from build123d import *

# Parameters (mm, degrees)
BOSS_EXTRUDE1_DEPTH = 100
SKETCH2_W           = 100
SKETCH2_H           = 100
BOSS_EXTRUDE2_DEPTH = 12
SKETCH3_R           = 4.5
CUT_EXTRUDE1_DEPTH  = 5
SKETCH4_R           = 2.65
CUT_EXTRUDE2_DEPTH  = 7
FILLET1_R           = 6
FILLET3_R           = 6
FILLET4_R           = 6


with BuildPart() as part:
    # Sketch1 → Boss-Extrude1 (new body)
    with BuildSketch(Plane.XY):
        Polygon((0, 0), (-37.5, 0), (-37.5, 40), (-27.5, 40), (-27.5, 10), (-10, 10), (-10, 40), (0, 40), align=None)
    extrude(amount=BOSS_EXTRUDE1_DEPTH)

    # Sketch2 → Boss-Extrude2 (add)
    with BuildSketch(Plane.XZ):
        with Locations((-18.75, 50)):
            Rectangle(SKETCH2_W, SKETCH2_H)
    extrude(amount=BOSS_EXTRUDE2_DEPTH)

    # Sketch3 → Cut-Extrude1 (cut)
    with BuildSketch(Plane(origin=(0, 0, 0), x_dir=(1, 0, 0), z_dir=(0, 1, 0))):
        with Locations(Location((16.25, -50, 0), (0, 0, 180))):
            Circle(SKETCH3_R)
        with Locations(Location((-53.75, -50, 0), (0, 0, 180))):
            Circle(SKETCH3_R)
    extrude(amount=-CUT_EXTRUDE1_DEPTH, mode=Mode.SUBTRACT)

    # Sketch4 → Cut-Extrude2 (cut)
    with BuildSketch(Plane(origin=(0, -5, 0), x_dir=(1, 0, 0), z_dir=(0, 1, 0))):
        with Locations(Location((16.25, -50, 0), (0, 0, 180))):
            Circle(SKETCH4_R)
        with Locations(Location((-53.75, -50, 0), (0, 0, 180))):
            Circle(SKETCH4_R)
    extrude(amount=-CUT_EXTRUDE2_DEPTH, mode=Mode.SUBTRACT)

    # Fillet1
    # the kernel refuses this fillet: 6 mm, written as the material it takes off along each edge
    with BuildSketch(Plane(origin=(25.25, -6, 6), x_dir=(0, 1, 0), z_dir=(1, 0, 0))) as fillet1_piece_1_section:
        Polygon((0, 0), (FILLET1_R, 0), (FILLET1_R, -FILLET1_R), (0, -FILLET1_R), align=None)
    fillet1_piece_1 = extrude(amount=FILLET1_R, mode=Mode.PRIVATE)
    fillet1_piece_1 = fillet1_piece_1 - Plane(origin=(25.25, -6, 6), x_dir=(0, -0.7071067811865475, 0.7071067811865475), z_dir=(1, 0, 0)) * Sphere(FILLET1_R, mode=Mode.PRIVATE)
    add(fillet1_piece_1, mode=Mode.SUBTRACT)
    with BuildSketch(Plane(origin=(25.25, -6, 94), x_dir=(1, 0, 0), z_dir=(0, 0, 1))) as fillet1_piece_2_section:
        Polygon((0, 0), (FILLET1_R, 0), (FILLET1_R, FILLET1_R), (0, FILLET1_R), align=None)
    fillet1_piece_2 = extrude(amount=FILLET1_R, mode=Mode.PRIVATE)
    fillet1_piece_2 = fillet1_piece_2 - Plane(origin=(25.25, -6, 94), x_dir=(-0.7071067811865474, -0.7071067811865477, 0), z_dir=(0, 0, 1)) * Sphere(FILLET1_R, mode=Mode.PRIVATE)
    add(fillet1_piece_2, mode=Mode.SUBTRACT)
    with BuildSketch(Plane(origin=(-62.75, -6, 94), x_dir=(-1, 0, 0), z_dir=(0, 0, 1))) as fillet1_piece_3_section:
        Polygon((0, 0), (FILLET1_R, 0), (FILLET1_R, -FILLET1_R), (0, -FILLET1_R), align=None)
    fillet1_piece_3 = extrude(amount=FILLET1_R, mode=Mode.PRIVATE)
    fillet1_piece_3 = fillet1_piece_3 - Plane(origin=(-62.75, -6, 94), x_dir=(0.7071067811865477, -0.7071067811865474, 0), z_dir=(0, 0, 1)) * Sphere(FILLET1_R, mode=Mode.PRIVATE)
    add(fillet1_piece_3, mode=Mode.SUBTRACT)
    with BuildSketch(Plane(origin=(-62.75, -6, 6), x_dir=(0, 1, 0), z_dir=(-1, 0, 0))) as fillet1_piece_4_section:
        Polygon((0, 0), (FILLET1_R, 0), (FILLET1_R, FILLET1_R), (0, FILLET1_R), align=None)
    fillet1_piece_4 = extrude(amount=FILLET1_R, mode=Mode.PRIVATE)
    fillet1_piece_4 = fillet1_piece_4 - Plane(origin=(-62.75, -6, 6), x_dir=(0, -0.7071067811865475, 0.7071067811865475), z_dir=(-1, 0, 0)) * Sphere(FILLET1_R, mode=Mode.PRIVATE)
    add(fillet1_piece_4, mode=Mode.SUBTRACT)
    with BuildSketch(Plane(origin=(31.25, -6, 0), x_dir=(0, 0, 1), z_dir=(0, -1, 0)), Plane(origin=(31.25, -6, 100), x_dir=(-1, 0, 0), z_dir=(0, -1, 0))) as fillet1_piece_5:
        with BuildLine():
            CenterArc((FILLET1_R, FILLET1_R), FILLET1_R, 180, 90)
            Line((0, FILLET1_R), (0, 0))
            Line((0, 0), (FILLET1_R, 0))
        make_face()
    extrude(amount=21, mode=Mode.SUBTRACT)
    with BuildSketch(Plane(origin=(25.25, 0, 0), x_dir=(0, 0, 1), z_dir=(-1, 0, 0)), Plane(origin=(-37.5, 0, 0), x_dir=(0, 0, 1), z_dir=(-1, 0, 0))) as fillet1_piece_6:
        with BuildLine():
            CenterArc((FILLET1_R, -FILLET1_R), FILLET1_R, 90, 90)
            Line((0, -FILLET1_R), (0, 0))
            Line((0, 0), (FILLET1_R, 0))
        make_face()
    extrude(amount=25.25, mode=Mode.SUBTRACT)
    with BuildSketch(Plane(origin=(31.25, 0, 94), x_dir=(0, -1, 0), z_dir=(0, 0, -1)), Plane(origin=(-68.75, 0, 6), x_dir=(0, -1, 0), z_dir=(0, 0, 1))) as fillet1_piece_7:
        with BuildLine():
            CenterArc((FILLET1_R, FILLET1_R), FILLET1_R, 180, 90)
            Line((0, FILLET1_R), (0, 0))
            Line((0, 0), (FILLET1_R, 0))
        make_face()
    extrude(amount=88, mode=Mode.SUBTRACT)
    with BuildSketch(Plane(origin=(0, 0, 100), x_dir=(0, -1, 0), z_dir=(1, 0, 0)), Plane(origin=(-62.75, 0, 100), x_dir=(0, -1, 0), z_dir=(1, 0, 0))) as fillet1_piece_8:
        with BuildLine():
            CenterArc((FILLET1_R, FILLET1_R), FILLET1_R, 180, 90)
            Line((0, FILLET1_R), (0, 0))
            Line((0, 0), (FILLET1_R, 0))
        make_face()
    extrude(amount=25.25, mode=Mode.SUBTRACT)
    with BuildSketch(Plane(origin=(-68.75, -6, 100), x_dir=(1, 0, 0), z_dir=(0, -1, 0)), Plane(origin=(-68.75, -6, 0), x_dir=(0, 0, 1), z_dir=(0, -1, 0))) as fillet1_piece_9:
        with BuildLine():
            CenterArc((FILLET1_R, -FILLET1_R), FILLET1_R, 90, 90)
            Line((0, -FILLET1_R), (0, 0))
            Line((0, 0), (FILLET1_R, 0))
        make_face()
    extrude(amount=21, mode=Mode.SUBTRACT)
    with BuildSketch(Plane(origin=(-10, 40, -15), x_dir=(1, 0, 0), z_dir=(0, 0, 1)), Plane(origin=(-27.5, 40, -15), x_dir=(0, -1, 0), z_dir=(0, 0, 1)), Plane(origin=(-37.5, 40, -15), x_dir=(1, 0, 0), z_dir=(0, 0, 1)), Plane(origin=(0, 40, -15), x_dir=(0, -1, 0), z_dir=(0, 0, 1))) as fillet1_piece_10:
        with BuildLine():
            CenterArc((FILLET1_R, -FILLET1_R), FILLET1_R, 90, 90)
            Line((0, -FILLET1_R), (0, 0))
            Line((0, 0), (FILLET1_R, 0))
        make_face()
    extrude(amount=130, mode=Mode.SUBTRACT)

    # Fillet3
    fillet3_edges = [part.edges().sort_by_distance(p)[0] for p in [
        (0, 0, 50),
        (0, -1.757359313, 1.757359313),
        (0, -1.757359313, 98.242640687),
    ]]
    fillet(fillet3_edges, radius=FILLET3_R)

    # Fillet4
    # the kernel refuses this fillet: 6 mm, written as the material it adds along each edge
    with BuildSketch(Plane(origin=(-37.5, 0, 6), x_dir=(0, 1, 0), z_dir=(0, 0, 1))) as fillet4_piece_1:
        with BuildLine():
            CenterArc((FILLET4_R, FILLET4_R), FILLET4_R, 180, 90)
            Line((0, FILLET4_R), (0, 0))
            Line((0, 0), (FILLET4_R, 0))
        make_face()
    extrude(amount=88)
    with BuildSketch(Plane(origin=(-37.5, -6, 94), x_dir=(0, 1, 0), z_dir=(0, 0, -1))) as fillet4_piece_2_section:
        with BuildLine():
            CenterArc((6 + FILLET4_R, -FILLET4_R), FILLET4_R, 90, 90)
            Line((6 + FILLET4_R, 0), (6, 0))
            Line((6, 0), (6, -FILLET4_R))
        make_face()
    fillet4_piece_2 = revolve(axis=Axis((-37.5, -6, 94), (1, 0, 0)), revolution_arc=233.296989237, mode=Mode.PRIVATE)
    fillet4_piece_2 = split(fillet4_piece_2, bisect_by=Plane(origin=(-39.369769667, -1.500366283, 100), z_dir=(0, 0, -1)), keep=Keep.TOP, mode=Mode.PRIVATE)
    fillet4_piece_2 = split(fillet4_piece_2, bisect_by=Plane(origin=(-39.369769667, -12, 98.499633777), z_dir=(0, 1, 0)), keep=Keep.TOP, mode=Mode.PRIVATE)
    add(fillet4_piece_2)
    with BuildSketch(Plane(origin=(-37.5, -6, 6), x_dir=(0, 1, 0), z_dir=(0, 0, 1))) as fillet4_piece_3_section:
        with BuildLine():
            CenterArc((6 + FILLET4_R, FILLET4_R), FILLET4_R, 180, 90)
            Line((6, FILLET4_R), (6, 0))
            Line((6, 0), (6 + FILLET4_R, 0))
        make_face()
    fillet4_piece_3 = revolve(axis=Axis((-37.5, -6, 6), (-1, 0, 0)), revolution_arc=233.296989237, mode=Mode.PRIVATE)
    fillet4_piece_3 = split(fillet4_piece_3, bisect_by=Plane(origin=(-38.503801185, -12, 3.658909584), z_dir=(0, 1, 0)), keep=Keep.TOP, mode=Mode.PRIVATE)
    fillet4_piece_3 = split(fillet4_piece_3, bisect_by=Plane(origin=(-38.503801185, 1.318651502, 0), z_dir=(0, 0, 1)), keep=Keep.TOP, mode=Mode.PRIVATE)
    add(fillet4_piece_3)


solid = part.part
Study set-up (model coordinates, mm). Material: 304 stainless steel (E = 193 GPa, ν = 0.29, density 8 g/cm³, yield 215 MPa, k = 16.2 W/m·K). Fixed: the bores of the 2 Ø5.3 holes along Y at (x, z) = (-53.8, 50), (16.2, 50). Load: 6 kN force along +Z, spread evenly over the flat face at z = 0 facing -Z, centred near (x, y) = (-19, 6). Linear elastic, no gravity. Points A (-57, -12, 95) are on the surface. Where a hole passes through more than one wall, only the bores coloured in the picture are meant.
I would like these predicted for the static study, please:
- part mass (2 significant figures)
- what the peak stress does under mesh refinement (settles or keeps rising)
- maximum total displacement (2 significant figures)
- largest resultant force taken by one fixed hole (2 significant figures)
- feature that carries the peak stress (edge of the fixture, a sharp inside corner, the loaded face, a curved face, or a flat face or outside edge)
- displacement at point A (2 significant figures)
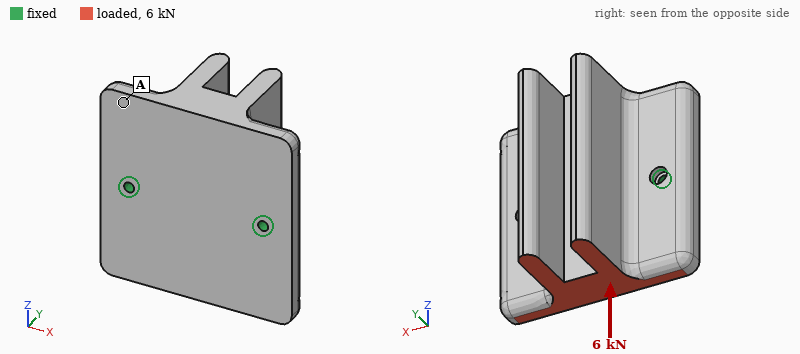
1.7 kg
keeps rising
77 µm
3.0 kN
edge of the fixture
47 µm
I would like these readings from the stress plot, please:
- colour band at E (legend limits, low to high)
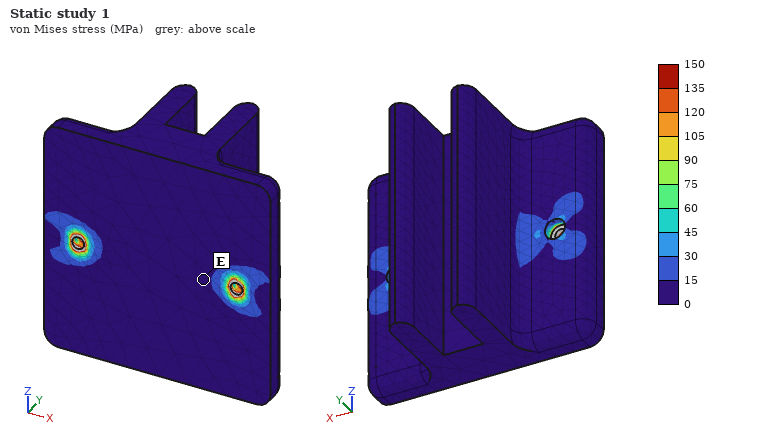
0 to 15 MPa
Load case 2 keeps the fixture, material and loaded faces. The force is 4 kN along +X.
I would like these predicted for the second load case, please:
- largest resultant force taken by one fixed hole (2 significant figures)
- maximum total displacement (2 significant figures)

3.5 kN
16 µm
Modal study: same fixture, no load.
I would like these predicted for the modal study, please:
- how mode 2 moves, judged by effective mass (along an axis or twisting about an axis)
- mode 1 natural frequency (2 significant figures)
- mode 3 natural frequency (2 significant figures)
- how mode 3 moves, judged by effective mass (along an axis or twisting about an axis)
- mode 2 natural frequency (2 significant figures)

along Y
1000 Hz
4500 Hz
along X
4100 Hz
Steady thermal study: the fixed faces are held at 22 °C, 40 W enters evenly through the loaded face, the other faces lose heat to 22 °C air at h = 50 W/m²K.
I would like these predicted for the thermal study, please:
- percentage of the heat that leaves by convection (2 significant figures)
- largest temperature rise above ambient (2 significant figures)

76 %
56 K
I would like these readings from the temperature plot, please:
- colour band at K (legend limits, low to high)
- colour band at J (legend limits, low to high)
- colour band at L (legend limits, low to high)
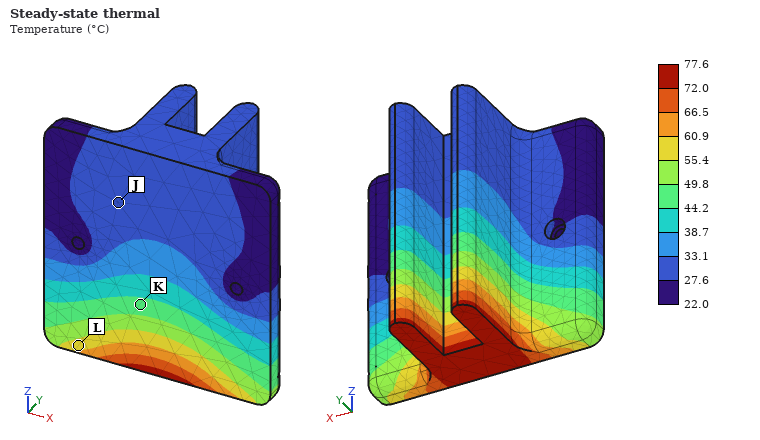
44.2 to 49.8 °C
27.6 to 33.1 °C
55.4 to 60.9 °C
